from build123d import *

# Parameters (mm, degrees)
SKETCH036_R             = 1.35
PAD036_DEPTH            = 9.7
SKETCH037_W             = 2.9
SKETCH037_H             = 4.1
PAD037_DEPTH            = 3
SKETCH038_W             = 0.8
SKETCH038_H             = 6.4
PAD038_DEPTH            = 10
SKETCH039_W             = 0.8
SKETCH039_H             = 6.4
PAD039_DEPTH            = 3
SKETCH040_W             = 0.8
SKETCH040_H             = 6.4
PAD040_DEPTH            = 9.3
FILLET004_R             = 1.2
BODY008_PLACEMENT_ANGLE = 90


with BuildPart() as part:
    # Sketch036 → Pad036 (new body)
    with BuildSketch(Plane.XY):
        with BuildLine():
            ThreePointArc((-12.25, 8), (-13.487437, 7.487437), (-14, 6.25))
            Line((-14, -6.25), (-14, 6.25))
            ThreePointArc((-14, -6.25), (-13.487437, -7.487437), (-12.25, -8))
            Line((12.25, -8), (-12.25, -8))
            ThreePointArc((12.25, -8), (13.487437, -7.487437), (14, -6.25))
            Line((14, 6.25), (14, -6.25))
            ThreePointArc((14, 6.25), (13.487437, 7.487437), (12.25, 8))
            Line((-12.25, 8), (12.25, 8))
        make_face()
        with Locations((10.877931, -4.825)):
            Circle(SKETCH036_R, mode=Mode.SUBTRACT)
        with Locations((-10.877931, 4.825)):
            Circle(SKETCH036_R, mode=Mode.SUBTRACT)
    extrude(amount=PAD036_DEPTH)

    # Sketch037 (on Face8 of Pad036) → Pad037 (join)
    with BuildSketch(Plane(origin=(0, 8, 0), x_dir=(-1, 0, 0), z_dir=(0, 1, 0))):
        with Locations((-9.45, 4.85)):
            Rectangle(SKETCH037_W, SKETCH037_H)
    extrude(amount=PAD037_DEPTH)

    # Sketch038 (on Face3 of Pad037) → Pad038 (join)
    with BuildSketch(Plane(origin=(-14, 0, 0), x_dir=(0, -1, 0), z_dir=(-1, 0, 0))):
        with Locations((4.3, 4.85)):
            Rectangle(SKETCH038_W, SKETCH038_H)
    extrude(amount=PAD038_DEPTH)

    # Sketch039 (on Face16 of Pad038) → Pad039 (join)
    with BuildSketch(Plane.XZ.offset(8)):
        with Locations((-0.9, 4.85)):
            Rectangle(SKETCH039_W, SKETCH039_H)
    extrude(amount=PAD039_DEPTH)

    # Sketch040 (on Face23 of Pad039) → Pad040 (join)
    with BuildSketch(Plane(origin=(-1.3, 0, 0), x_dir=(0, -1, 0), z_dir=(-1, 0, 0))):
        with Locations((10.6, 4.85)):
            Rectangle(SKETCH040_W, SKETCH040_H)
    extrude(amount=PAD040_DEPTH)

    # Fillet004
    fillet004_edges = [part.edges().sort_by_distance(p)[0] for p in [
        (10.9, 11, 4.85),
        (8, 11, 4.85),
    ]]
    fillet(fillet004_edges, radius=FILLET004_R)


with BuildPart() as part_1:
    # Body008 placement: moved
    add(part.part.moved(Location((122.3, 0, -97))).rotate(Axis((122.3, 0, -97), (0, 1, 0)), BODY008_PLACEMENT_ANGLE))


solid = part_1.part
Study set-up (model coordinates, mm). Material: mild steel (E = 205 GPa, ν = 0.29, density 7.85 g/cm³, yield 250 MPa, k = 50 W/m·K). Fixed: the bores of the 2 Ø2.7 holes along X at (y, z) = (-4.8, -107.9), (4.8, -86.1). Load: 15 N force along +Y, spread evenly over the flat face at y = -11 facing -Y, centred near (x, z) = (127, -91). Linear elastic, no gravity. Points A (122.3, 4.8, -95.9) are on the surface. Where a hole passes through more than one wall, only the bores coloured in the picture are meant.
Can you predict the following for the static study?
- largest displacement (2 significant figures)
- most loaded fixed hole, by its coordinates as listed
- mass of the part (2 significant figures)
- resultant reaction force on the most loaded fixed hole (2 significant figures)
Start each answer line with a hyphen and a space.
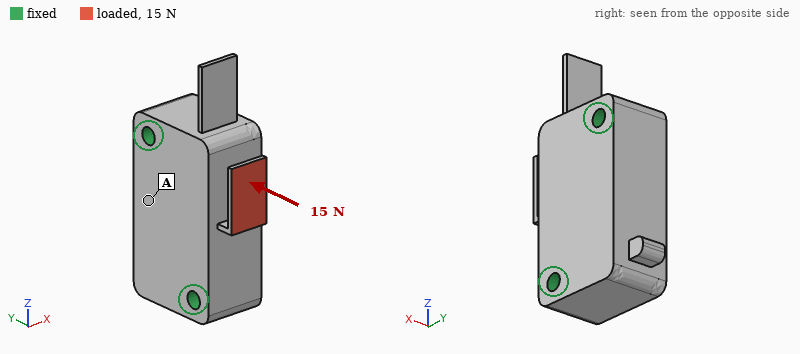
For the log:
- 55 µm
- (4.8, -86.1)
- 34 g
- 12 N
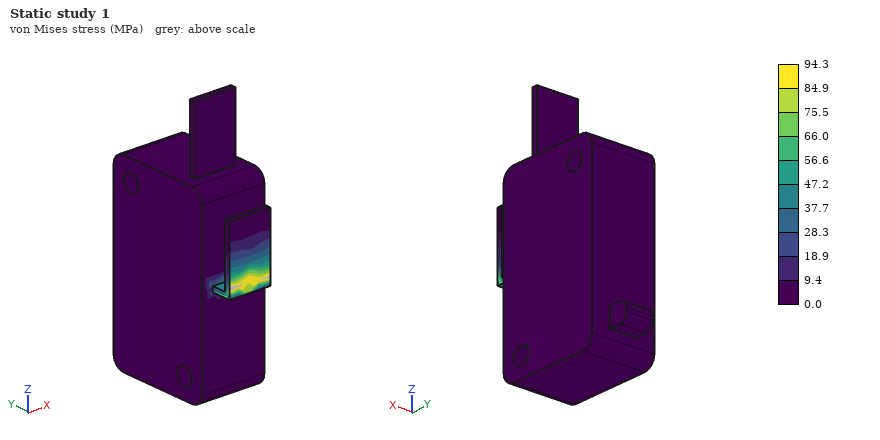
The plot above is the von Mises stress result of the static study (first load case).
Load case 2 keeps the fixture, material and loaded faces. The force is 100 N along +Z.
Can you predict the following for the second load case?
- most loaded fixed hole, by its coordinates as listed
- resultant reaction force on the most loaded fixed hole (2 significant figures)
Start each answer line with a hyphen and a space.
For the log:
- (-4.8, -107.9)
- 78 N
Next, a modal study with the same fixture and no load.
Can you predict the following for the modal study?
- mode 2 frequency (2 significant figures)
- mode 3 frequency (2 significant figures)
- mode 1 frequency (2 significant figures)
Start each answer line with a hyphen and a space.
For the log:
- 6400 Hz
- 12 kHz
- 5100 Hz
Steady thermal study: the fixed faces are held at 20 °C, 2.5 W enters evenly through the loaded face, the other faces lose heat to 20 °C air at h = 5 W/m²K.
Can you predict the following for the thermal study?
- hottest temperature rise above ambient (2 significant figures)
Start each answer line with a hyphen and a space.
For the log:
- 75 K
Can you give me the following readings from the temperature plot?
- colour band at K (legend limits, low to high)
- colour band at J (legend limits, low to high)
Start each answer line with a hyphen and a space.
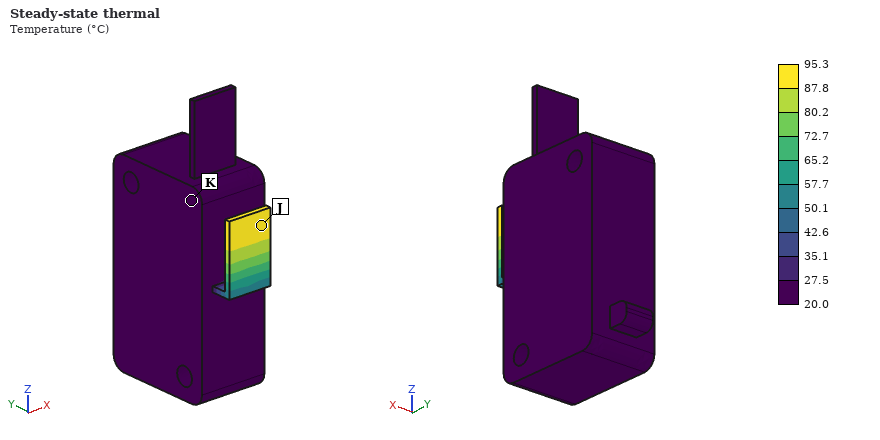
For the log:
- 20.0 to 27.5 °C
- 87.8 to 95.3 °C
